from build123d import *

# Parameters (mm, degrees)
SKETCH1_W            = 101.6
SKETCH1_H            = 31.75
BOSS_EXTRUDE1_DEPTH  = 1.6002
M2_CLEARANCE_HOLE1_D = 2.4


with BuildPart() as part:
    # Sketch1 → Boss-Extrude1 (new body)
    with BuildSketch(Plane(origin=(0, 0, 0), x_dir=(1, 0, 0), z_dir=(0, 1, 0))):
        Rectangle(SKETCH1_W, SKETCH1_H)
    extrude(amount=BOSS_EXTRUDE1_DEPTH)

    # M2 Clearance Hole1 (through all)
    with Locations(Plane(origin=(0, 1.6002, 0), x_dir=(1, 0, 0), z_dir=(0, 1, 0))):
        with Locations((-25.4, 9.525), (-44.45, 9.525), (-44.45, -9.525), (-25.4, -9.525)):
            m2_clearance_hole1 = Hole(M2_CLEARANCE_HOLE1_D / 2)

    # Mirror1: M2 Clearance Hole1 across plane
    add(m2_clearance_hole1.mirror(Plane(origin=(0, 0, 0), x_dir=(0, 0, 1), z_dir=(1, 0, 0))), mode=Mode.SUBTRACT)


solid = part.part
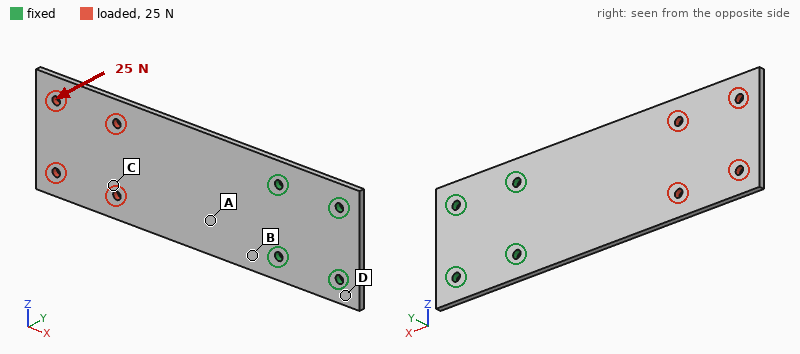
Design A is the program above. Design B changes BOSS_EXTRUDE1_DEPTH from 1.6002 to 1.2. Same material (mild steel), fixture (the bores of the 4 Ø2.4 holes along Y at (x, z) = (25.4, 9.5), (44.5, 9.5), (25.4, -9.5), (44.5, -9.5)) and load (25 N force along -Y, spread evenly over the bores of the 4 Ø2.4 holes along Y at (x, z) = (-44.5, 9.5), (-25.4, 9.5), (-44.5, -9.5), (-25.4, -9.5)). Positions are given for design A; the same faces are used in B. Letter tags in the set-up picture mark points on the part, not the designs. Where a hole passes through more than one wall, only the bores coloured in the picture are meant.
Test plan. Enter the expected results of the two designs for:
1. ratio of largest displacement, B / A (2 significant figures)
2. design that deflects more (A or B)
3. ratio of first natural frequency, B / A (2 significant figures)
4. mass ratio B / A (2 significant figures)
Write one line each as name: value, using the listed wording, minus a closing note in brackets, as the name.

ratio of largest displacement, B / A: 2.4
design that deflects more: B
ratio of first natural frequency, B / A: 0.75
mass ratio B / A: 0.75
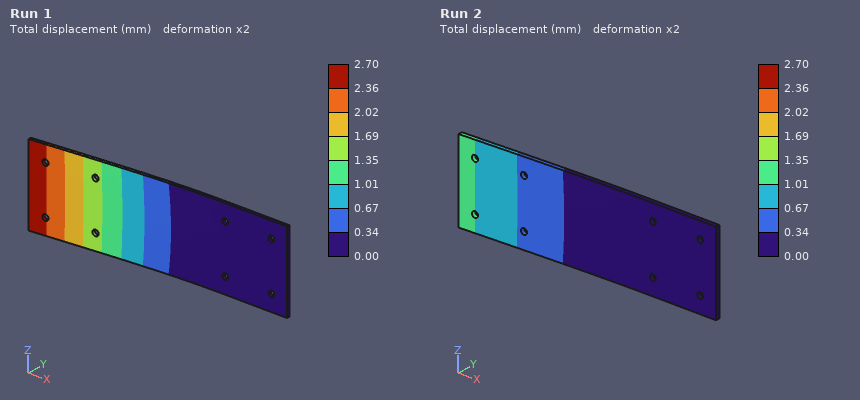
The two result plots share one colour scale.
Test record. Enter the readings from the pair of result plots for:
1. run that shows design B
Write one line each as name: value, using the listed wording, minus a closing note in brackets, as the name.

run that shows design B: Run 1
